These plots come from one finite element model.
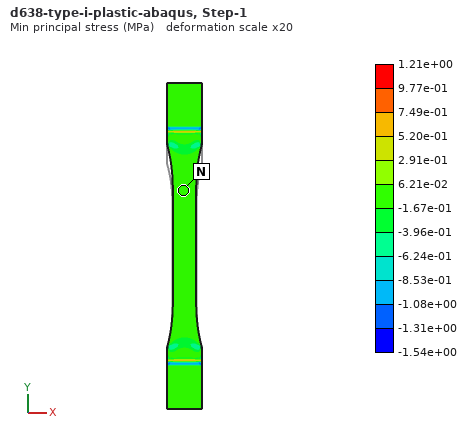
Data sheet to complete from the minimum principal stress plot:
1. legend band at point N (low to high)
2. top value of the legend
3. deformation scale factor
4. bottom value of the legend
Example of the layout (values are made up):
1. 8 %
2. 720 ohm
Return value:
1. -1.67e-01 to 6.21e-02 MPa
2. 1.21e+00 MPa
3. 20
4. -1.54e+00 MPa
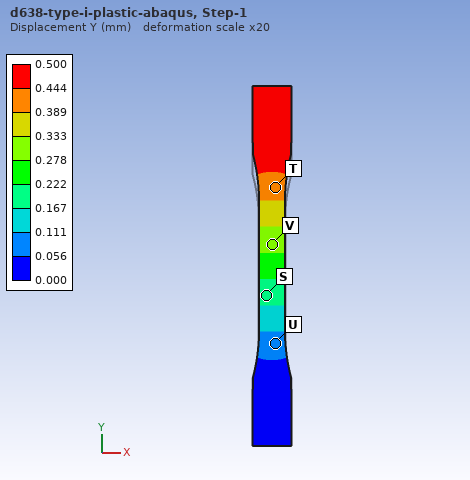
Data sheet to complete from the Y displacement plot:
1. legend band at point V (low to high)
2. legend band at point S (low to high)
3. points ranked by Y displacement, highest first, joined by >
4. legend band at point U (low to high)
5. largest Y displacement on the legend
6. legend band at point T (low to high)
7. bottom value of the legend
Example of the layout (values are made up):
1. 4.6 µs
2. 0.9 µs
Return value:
1. 0.278 to 0.333 mm
2. 0.167 to 0.222 mm
3. T > V > S > U
4. 0.056 to 0.111 mm
5. 0.500 mm
6. 0.389 to 0.444 mm
7. 0.000 mm
